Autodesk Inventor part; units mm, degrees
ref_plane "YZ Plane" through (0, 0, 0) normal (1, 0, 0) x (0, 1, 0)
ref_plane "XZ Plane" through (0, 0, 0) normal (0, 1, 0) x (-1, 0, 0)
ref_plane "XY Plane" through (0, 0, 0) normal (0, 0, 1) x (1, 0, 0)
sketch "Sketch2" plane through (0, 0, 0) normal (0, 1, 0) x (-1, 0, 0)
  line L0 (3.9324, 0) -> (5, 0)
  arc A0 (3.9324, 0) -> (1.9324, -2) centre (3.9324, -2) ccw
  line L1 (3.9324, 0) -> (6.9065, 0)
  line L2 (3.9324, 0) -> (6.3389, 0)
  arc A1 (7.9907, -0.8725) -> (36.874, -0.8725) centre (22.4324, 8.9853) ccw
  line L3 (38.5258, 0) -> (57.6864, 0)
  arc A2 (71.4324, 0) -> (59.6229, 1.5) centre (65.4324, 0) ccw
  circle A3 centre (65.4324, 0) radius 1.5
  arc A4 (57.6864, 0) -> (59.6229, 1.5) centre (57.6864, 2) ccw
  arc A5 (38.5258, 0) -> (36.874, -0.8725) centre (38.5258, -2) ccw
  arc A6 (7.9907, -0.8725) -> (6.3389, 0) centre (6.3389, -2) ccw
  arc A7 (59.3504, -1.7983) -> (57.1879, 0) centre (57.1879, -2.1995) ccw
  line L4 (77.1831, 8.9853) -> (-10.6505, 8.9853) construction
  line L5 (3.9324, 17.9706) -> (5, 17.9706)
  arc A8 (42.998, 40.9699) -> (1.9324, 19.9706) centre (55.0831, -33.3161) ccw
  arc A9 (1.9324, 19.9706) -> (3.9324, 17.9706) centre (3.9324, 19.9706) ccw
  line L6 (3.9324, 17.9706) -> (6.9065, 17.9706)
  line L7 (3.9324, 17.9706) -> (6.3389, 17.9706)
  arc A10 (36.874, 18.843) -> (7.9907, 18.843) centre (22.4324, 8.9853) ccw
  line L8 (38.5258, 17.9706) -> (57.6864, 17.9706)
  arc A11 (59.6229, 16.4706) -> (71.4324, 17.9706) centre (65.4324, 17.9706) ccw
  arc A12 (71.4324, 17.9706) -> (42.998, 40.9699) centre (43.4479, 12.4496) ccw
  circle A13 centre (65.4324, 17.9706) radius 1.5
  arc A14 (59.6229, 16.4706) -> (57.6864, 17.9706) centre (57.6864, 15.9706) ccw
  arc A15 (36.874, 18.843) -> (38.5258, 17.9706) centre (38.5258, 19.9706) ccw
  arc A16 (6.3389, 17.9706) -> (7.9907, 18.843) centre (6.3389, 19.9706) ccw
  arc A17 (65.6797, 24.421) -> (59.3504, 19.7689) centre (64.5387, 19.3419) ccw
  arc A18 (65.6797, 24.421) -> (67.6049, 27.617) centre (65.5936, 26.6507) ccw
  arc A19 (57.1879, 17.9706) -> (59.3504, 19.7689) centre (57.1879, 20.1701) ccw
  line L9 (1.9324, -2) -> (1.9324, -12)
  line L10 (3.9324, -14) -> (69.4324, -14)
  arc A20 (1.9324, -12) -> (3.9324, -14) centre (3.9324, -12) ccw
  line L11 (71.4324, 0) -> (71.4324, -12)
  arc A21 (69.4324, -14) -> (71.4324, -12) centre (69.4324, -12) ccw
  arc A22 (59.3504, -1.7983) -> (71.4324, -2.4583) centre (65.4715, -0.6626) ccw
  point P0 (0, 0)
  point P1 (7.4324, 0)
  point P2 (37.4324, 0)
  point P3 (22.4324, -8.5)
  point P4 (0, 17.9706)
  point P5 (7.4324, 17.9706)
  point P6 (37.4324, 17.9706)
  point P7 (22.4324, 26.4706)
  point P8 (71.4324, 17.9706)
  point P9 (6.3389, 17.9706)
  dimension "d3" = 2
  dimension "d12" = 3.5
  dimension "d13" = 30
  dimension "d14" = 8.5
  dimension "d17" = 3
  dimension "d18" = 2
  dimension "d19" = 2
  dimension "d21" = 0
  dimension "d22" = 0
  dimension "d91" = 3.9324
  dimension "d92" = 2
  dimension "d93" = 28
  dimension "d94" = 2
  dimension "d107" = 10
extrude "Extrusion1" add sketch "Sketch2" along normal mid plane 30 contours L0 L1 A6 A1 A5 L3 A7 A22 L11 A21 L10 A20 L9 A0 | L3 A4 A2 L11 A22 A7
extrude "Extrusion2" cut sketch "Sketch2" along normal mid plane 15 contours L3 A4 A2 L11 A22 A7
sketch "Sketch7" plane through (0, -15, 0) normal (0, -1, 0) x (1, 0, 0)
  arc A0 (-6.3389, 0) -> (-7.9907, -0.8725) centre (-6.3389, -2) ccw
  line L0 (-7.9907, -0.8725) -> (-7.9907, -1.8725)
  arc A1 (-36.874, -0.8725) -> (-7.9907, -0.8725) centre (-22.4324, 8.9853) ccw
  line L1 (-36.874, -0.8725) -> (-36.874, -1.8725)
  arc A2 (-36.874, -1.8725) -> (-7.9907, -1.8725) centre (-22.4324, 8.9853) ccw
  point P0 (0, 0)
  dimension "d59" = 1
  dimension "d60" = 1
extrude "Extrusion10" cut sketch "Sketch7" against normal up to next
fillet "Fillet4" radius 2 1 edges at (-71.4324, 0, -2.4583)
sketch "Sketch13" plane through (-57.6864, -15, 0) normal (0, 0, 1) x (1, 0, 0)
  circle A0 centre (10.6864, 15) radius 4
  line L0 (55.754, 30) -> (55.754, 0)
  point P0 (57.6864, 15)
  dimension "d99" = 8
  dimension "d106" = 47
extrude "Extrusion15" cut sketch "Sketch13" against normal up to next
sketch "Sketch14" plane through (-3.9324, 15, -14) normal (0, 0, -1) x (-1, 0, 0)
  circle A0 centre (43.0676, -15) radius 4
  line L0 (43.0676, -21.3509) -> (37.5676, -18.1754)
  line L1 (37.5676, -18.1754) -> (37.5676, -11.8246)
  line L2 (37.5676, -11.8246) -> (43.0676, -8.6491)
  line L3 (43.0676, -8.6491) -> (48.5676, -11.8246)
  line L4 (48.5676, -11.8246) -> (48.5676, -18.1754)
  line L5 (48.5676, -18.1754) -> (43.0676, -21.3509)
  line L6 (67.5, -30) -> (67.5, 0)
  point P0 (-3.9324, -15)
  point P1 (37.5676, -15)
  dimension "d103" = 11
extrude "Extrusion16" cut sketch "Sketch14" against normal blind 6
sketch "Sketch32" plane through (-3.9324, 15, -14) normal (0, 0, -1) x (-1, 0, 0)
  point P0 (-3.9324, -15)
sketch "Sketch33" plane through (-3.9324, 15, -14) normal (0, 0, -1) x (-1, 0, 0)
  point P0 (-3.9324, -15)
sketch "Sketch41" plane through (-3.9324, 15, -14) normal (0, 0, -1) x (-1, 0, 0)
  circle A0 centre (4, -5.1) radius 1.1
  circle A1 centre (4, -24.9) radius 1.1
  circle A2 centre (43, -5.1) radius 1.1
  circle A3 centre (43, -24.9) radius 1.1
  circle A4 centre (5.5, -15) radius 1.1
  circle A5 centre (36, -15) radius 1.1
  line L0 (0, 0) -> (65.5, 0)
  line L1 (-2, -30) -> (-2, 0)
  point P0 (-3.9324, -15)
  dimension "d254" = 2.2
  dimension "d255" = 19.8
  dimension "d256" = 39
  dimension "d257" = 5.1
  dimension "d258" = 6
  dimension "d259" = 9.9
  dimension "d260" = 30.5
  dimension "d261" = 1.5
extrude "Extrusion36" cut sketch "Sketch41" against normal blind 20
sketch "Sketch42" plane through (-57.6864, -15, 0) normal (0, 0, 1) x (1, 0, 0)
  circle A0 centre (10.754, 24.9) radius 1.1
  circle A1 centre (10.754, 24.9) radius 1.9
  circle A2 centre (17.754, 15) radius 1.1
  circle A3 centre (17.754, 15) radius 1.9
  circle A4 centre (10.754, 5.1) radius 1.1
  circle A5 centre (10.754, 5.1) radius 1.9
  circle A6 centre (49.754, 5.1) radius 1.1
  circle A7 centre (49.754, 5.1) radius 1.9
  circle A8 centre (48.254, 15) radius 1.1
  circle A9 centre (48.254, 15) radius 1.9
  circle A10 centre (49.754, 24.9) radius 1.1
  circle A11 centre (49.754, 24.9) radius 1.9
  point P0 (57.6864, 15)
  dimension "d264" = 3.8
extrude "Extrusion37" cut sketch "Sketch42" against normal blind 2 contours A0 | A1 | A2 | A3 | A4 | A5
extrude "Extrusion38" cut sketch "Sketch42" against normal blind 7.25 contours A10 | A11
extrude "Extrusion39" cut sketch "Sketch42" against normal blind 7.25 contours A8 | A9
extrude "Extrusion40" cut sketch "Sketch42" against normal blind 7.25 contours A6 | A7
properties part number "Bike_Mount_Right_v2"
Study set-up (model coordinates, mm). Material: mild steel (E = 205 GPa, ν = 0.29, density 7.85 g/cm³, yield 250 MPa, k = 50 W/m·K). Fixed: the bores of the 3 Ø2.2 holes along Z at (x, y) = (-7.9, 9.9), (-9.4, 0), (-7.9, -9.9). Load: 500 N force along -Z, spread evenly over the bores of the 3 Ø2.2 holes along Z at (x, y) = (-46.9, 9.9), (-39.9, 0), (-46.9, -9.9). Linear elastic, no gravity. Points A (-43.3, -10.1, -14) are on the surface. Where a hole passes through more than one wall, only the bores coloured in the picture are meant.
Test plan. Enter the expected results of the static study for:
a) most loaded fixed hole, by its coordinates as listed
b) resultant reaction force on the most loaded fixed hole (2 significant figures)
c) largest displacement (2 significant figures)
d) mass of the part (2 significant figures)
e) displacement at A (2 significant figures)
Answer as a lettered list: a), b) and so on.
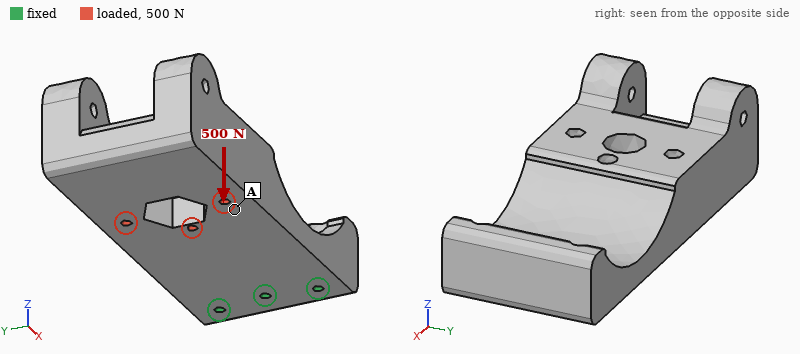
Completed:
a) (-9.4, 0)
b) 610 N
c) 0.15 mm
d) 170 g
e) 0.068 mm
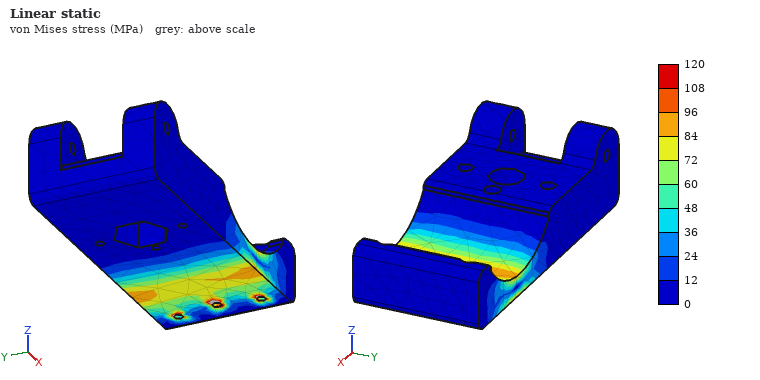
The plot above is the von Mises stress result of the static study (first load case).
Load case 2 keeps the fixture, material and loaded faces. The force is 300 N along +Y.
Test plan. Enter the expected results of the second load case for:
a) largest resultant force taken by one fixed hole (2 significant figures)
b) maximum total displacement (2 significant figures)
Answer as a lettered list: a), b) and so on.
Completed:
a) 520 N
b) 6.7 µm
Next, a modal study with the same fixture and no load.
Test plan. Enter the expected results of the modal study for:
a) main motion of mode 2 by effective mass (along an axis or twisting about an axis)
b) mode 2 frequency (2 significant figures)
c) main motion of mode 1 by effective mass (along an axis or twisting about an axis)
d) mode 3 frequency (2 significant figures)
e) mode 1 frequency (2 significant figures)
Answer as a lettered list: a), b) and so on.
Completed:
a) along Y
b) 3200 Hz
c) along Z
d) 4400 Hz
e) 880 Hz
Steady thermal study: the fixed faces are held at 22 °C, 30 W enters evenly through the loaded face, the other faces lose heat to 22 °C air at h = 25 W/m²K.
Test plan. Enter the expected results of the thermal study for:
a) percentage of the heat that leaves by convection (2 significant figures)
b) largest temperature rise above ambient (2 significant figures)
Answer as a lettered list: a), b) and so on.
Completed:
a) 32 %
b) 78 K
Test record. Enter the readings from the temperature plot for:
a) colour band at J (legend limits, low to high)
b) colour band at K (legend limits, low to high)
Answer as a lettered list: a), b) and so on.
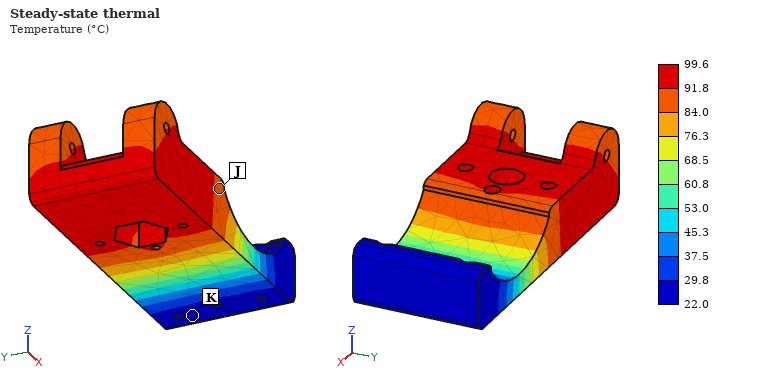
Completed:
a) 84.0 to 91.8 °C
b) 22.0 to 29.8 °C
